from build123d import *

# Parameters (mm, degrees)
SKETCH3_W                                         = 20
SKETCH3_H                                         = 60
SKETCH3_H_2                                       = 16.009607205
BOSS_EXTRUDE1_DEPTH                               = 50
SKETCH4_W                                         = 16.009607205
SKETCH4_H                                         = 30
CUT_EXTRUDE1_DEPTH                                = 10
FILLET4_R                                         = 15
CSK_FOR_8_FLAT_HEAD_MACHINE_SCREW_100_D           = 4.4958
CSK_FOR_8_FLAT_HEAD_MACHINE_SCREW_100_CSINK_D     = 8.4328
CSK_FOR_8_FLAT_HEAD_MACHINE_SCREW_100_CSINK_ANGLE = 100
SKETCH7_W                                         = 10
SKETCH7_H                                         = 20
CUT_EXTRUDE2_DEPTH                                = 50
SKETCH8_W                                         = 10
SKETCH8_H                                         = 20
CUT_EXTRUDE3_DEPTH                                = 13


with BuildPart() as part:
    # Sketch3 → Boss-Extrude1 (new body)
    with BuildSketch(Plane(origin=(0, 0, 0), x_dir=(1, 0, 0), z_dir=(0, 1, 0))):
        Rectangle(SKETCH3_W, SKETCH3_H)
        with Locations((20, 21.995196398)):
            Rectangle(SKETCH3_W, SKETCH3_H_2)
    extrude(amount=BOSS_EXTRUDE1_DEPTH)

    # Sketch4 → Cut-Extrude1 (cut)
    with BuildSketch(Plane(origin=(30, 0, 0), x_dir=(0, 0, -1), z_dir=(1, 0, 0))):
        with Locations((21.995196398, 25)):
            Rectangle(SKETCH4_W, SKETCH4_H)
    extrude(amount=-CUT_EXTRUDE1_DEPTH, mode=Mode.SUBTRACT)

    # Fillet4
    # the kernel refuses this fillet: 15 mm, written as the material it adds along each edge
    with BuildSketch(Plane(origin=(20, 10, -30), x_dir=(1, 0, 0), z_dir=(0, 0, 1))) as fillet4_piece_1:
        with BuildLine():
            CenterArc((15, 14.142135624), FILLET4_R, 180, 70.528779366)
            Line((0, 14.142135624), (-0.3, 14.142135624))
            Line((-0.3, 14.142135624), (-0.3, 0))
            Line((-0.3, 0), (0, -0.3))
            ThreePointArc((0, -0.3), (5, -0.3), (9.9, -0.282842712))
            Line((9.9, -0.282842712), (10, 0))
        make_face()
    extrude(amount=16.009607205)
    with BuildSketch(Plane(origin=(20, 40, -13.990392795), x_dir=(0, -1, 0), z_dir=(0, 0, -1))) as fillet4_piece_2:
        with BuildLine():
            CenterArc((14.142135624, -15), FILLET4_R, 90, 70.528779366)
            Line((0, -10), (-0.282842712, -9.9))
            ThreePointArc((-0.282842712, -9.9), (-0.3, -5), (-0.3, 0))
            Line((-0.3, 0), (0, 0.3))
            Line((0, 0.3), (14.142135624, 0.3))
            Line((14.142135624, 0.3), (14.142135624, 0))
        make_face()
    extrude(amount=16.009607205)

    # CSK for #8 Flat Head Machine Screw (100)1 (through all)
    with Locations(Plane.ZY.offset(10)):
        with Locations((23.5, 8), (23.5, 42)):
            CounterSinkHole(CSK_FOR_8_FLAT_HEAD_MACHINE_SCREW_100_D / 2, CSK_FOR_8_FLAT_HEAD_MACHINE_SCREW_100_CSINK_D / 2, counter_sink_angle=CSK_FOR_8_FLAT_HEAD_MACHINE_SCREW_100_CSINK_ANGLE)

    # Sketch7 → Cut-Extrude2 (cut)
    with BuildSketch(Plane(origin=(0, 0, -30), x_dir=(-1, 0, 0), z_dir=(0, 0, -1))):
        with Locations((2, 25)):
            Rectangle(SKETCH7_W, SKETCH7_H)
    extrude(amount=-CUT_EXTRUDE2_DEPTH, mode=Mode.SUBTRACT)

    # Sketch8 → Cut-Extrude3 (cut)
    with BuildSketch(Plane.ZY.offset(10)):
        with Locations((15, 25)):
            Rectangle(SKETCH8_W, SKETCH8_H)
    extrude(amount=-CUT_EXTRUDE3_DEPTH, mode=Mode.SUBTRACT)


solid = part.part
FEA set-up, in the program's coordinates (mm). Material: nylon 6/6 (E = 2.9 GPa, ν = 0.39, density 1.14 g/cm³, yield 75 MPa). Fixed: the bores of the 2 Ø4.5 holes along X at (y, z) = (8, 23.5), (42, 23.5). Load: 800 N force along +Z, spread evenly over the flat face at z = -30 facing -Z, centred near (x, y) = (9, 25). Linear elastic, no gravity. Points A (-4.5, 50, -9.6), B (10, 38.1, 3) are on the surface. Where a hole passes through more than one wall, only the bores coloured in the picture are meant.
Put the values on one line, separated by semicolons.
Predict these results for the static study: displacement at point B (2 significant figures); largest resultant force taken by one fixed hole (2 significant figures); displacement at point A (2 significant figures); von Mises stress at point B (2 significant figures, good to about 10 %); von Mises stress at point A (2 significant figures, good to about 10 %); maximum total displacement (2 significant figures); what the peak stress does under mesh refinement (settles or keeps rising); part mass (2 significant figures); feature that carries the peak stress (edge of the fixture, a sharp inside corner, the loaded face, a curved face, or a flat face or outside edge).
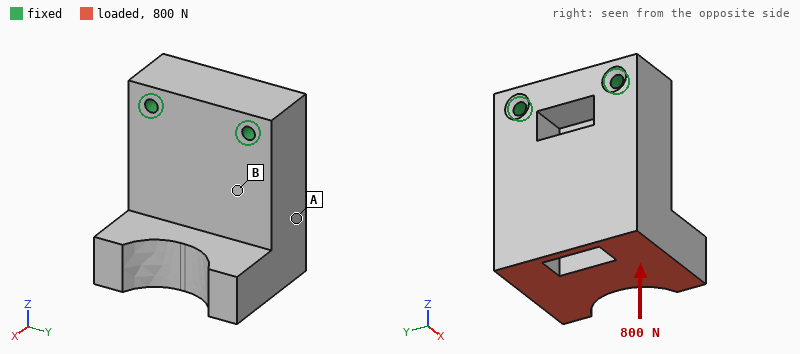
0.042 mm; 410 N; 0.058 mm; 3.2 MPa; 0.70 MPa; 0.23 mm; keeps rising; 70 g; edge of the fixture
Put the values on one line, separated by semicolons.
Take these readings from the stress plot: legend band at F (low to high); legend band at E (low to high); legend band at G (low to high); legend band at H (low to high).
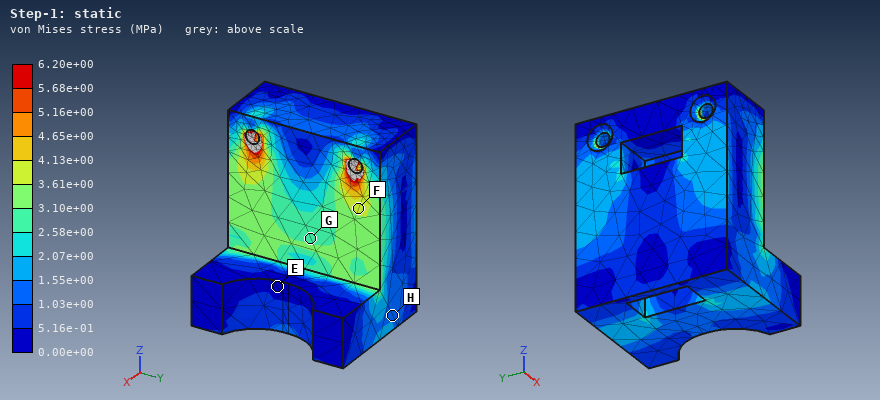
3.61e+00 to 4.13e+00 MPa; 0.00e+00 to 5.16e-01 MPa; 2.58e+00 to 3.10e+00 MPa; 1.03e+00 to 1.55e+00 MPa
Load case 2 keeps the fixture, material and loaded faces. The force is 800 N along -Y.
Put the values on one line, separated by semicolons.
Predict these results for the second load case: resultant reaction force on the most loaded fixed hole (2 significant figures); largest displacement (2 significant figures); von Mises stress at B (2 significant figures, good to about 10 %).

1.2 kN; 0.23 mm; 4.1 MPa
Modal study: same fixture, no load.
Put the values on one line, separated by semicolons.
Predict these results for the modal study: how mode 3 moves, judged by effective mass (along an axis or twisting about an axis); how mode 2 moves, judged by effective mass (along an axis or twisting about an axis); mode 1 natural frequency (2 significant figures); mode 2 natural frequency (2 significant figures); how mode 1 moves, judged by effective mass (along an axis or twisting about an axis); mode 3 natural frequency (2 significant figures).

along Y; along Y; 1000 Hz; 1900 Hz; along X; 2200 Hz
